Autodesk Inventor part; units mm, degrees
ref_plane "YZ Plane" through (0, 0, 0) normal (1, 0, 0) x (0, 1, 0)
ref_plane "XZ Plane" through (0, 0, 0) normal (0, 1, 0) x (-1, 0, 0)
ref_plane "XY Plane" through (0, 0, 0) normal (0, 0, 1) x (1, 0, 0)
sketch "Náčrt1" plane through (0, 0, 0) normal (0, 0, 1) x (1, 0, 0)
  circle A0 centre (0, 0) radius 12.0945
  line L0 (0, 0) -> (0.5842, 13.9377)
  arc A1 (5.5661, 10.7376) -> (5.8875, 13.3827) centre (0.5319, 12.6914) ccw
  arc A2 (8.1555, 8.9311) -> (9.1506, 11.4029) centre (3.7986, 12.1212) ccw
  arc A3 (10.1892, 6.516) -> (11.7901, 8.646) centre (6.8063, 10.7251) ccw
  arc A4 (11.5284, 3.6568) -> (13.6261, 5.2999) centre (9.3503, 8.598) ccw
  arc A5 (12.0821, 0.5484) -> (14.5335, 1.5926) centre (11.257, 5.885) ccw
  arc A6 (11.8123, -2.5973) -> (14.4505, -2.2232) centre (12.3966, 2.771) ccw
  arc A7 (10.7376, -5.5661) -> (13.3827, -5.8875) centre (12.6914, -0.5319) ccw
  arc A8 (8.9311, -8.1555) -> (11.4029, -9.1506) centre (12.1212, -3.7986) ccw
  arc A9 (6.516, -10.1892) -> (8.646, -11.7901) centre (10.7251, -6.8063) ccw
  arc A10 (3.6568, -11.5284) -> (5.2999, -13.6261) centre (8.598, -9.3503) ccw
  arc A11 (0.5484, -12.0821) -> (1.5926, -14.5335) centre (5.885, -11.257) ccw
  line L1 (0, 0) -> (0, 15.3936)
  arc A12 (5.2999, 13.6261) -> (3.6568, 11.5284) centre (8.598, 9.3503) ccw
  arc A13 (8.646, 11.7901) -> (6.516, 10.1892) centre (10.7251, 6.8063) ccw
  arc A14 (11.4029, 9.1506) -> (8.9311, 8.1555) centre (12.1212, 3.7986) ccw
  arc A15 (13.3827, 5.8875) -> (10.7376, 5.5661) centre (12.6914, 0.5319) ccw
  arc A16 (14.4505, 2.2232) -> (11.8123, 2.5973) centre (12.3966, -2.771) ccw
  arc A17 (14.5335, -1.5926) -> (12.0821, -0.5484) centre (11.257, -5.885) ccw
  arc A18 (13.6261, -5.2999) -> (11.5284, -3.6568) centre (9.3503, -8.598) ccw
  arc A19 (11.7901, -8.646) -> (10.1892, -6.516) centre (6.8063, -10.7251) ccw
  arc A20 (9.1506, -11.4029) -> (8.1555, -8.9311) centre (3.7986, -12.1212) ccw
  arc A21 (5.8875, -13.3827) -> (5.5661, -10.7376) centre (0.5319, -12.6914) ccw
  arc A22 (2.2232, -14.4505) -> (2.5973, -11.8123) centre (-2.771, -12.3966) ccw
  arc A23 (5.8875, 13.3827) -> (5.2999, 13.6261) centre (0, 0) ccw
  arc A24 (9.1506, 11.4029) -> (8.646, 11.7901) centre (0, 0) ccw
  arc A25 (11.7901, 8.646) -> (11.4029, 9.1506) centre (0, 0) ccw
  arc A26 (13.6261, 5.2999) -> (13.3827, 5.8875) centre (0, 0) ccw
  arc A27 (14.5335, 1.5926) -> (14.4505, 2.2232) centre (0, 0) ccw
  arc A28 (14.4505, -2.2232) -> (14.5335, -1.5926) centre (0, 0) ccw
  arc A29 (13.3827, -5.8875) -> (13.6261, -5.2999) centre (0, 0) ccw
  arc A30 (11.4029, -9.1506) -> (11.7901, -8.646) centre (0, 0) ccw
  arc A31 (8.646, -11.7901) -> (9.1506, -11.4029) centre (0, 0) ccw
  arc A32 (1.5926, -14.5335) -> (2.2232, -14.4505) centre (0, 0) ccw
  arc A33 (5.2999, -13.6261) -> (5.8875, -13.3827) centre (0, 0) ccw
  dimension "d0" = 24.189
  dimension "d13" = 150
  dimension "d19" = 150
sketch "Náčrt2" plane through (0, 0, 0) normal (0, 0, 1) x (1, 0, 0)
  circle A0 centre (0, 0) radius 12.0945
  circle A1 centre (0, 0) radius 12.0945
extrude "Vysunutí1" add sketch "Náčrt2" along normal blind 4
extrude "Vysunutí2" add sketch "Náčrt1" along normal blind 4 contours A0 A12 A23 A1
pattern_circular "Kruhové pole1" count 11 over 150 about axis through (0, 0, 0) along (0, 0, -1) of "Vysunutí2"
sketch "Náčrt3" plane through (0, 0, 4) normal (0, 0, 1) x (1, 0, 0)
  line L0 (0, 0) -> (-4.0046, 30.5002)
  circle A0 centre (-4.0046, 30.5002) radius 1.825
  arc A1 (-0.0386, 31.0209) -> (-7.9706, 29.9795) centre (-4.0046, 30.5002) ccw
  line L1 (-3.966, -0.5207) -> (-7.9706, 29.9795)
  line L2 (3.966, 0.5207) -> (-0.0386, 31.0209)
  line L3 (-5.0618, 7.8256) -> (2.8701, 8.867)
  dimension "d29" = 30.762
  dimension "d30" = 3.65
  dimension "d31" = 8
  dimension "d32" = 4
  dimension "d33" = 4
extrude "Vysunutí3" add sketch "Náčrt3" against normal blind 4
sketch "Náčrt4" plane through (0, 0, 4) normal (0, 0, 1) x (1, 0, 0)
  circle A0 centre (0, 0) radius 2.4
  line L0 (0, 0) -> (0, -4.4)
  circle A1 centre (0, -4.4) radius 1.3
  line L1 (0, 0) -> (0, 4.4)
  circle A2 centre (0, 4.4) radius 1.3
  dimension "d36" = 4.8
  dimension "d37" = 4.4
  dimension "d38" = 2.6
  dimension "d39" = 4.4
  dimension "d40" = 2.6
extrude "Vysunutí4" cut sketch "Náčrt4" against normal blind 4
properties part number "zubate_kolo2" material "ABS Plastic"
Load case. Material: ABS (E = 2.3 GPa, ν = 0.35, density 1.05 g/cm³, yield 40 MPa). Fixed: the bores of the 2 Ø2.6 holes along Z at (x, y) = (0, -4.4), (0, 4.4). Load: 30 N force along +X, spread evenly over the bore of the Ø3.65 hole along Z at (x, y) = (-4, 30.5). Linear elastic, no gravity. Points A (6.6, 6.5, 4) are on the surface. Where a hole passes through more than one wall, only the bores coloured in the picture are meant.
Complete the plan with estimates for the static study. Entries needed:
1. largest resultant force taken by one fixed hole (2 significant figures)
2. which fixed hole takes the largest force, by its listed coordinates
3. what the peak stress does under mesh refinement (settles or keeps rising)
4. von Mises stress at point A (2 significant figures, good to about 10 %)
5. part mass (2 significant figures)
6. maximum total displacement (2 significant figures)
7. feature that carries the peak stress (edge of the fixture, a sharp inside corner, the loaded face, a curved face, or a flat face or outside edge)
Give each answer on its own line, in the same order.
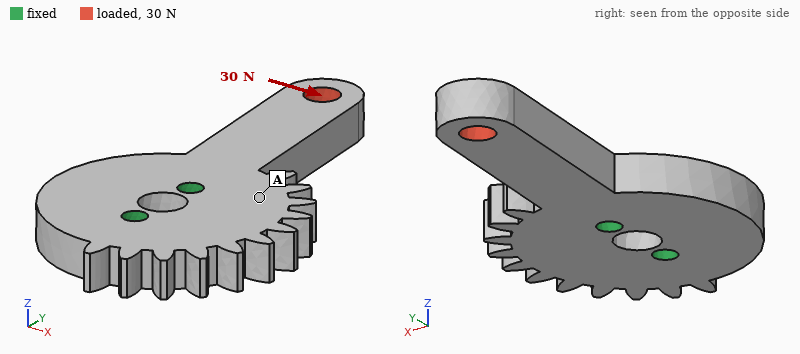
88 N
(0, 4.4)
keeps rising
2.0 MPa
2.7 g
0.44 mm
a sharp inside corner
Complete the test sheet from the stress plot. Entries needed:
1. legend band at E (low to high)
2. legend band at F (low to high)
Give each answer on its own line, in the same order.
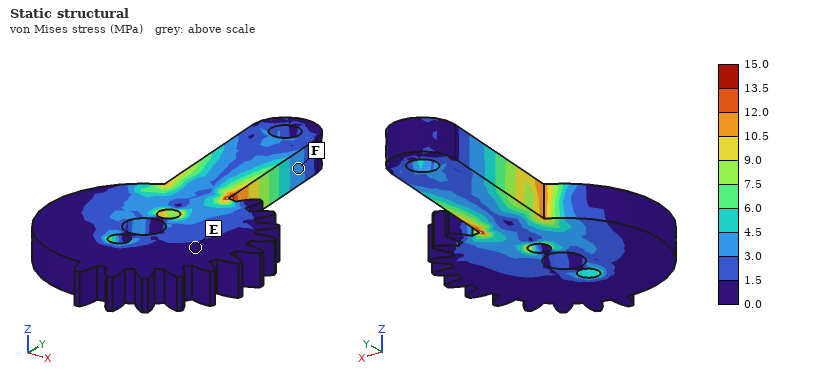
0.0 to 1.5 MPa
3.0 to 4.5 MPa
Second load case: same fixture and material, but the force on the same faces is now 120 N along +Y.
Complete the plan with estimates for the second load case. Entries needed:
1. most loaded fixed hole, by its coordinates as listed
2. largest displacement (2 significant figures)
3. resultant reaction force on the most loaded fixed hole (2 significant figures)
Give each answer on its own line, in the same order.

(0, 4.4)
0.24 mm
99 N
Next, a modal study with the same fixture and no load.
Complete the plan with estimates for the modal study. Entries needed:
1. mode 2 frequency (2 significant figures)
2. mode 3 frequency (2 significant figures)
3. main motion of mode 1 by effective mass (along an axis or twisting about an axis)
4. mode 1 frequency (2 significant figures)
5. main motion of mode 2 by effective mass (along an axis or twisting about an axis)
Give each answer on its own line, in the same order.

2700 Hz
5500 Hz
along Z
1300 Hz
along X
